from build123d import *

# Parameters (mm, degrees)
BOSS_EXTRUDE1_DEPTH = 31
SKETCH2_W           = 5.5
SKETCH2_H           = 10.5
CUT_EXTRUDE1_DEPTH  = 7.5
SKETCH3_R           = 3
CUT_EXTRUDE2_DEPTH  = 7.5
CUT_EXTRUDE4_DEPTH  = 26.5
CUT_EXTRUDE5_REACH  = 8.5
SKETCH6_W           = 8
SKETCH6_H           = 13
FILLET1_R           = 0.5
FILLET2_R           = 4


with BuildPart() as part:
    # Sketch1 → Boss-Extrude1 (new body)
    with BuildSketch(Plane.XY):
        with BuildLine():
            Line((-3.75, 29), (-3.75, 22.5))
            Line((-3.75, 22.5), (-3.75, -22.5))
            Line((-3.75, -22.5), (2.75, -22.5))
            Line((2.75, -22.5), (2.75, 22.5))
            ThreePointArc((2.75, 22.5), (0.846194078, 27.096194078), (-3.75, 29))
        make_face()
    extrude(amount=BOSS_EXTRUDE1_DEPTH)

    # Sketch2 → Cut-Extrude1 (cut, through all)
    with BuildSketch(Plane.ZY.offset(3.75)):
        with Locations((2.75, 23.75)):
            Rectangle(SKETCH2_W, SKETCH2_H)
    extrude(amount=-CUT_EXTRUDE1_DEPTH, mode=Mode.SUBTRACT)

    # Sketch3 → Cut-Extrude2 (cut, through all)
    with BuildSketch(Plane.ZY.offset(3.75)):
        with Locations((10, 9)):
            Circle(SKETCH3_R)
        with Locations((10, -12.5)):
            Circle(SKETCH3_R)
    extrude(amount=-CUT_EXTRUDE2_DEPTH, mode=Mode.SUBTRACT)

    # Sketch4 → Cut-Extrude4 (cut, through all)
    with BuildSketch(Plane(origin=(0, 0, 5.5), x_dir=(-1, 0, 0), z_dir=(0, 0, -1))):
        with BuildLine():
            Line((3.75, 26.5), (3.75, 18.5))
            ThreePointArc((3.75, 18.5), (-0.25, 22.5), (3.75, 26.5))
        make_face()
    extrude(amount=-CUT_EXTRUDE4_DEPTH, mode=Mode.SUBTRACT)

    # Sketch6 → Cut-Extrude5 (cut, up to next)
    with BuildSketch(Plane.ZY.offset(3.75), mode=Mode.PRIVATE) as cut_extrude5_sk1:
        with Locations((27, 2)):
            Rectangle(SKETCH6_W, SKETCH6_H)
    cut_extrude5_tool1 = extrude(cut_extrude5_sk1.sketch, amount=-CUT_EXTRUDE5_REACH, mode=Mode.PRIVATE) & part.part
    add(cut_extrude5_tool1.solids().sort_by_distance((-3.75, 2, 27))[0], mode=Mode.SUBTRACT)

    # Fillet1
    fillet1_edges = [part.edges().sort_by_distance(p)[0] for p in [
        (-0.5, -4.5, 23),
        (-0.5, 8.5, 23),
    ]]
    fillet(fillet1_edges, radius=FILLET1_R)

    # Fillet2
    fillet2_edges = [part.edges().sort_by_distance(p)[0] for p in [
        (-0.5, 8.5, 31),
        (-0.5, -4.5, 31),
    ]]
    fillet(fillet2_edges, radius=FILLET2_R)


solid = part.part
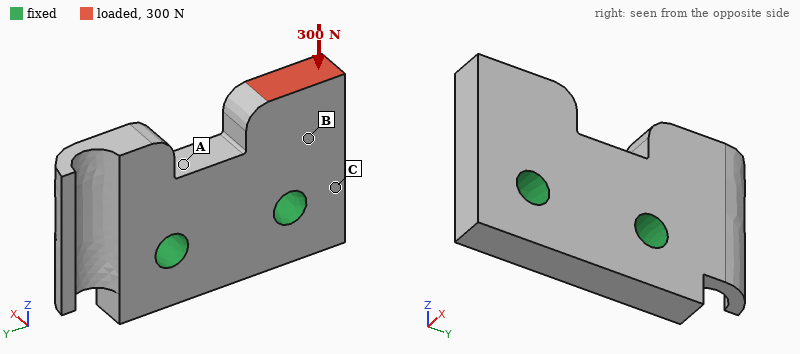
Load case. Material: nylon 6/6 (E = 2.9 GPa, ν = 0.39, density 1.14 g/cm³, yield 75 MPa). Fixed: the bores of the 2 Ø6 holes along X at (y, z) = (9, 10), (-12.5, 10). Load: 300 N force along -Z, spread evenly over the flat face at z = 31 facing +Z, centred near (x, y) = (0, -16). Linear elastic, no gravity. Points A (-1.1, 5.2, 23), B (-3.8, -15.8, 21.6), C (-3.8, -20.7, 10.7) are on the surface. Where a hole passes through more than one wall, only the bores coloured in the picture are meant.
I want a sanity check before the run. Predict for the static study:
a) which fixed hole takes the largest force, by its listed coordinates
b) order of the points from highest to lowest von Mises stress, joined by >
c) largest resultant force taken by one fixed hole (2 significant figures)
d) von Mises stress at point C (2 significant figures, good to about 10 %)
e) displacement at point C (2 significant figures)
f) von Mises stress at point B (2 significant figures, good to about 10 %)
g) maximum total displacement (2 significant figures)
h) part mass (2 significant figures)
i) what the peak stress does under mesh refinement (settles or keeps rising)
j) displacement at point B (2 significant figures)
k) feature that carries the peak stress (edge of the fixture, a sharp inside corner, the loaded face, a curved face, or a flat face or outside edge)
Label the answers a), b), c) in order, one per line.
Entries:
a) (-12.5, 10)
b) B > C > A
c) 320 N
d) 1.8 MPa
e) 11 µm
f) 3.6 MPa
g) 43 µm
h) 9.2 g
i) keeps rising
j) 18 µm
k) edge of the fixture
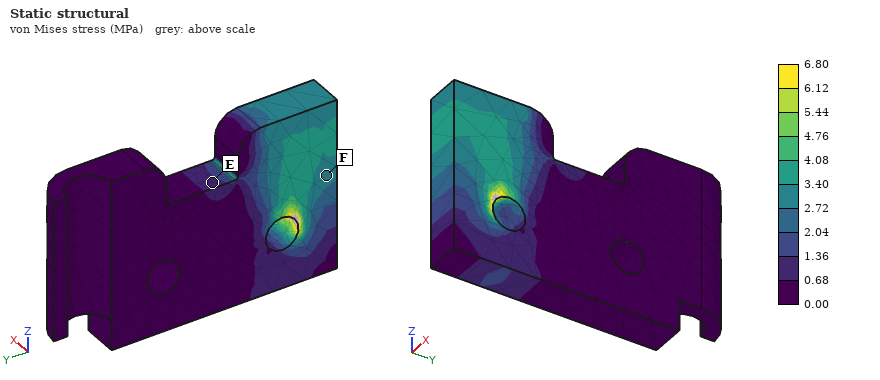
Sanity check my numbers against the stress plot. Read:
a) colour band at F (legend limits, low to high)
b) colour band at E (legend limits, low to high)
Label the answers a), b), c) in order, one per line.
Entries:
a) 2.72 to 3.40 MPa
b) 0.68 to 1.36 MPa
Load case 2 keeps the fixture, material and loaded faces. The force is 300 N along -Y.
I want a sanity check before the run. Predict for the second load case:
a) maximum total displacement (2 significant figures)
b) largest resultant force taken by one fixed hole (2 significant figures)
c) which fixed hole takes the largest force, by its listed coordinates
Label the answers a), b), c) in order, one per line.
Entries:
a) 0.13 mm
b) 290 N
c) (9, 10)
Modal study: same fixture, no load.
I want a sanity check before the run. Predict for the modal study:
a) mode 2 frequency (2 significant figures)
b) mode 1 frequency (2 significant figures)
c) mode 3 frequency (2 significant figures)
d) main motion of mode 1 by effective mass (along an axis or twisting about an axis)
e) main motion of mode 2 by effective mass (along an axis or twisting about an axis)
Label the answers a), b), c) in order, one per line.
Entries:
a) 4400 Hz
b) 3300 Hz
c) 5100 Hz
d) along X
e) along X
